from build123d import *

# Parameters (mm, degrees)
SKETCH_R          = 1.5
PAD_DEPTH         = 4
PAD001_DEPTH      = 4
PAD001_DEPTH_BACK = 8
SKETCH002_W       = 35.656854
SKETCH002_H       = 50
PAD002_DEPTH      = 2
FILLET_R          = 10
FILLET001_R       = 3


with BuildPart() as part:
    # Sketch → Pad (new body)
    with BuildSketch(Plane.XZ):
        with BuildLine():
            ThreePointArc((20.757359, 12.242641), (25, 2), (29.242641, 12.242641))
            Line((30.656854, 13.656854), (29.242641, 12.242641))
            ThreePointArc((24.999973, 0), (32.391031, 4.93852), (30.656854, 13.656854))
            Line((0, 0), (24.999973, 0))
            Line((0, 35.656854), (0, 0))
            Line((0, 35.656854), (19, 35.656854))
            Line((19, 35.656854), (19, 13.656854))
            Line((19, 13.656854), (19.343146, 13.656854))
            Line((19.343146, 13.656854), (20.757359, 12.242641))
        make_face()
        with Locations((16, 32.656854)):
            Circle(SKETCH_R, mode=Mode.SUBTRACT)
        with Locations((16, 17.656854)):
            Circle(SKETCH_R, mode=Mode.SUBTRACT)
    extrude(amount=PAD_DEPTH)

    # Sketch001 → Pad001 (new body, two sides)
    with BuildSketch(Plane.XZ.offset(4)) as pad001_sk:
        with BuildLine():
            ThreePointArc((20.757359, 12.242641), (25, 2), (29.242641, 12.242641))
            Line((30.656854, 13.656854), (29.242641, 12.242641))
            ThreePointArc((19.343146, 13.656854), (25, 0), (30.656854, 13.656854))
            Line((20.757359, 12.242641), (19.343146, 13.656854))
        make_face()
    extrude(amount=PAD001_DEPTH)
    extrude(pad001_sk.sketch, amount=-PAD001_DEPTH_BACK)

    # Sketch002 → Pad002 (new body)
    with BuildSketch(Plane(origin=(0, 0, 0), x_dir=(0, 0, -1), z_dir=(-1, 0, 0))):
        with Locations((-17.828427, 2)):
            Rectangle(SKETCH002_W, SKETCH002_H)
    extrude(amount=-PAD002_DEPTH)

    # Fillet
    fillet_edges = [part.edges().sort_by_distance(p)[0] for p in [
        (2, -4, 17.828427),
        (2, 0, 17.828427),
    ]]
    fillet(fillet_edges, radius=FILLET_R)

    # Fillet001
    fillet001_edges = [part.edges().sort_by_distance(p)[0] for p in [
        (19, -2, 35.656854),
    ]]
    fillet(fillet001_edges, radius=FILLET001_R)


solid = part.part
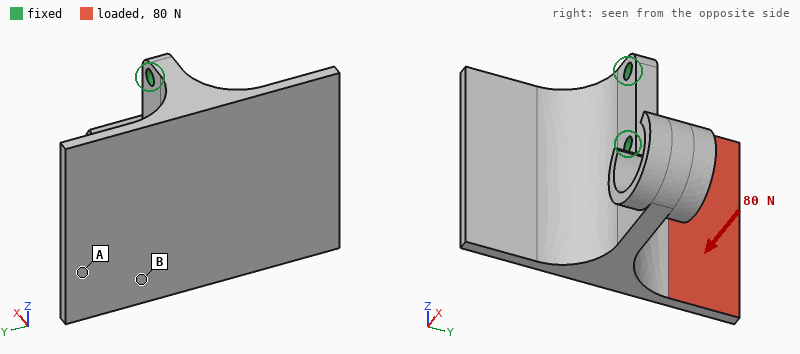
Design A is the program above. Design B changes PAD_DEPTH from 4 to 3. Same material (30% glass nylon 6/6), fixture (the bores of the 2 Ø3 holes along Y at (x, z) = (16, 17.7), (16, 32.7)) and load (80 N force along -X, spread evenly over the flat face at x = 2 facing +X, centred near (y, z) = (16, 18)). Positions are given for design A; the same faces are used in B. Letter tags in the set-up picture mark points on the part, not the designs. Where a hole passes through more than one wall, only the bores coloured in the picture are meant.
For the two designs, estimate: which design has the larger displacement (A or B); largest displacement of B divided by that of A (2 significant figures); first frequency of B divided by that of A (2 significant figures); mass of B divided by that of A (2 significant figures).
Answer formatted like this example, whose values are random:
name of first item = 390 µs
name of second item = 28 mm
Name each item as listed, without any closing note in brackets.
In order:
which design has the larger displacement = B
largest displacement of B divided by that of A = 1.5
first frequency of B divided by that of A = 0.72
mass of B divided by that of A = 0.93
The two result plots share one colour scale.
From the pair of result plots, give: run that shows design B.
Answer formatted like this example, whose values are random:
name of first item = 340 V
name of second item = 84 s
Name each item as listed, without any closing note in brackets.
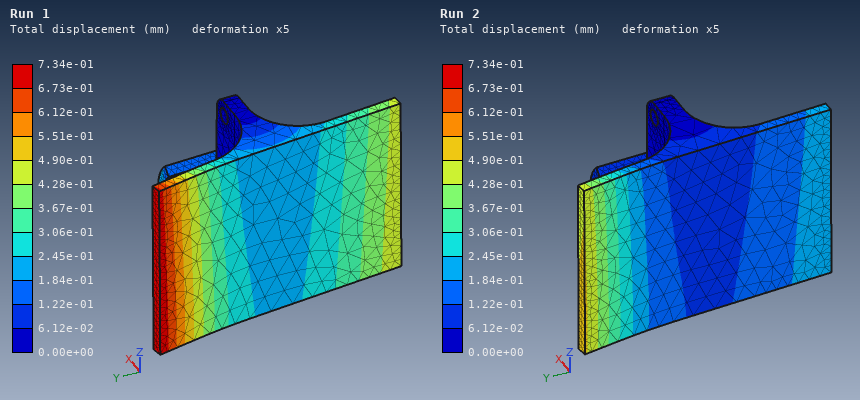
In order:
run that shows design B = Run 1
